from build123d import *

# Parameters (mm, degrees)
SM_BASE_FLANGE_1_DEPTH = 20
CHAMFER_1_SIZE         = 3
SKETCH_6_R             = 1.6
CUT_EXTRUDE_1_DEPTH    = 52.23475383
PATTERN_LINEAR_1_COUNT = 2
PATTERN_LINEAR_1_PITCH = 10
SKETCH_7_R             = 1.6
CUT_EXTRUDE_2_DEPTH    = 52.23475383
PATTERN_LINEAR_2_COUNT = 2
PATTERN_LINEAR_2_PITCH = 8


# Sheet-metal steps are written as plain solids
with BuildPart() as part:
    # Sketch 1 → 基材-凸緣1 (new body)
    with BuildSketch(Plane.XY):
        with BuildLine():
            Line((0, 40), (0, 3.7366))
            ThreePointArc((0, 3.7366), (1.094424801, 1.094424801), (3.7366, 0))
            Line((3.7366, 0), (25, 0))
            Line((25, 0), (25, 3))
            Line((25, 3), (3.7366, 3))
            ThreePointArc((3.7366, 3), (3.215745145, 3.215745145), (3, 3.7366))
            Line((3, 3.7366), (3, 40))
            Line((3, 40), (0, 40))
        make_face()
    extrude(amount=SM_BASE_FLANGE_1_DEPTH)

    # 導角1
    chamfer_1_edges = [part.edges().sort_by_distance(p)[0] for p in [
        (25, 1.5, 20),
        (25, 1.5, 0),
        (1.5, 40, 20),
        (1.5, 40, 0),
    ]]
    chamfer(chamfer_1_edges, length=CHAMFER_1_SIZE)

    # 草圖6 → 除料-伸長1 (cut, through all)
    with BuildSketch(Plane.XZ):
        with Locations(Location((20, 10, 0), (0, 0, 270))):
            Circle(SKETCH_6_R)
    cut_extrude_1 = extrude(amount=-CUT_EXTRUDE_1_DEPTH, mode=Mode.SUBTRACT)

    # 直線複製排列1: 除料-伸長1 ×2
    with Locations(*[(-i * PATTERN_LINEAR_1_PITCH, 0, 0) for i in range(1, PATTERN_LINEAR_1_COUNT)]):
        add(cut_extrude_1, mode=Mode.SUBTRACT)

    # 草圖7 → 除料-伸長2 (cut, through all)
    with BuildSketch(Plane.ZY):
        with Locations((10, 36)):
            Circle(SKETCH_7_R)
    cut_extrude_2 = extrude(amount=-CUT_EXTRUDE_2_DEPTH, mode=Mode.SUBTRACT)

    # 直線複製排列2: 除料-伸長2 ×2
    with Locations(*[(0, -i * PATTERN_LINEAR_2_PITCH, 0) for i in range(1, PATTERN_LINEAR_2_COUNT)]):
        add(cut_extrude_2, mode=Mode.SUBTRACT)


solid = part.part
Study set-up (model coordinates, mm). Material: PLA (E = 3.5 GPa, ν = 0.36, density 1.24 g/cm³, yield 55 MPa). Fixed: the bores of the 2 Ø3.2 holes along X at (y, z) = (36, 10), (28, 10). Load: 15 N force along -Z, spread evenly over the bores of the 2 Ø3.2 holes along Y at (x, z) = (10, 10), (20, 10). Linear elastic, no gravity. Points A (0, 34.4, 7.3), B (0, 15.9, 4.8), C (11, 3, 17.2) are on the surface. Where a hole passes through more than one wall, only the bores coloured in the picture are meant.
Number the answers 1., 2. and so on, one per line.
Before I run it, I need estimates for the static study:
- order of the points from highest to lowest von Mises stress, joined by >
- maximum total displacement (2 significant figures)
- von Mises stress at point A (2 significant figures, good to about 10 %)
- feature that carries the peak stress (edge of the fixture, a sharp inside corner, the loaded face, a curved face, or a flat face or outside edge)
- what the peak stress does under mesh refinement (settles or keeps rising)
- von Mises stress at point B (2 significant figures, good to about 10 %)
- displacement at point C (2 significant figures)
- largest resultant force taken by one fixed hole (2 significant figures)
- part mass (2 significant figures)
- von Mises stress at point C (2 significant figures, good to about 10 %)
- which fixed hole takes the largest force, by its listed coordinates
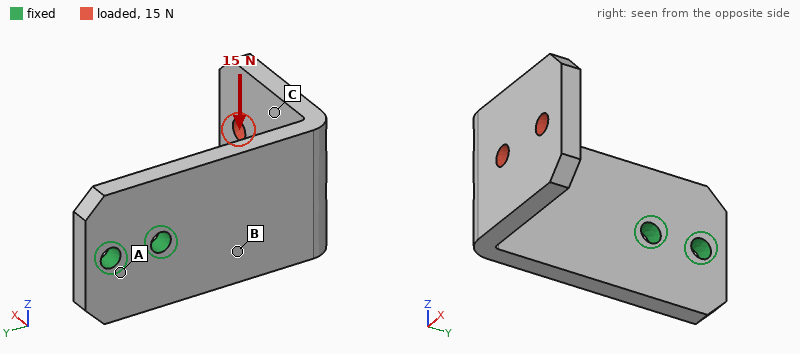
1. B > A > C
2. 0.60 mm
3. 3.1 MPa
4. edge of the fixture
5. keeps rising
6. 5.3 MPa
7. 0.30 mm
8. 47 N
9. 4.4 g
10. 1.2 MPa
11. (28, 10)
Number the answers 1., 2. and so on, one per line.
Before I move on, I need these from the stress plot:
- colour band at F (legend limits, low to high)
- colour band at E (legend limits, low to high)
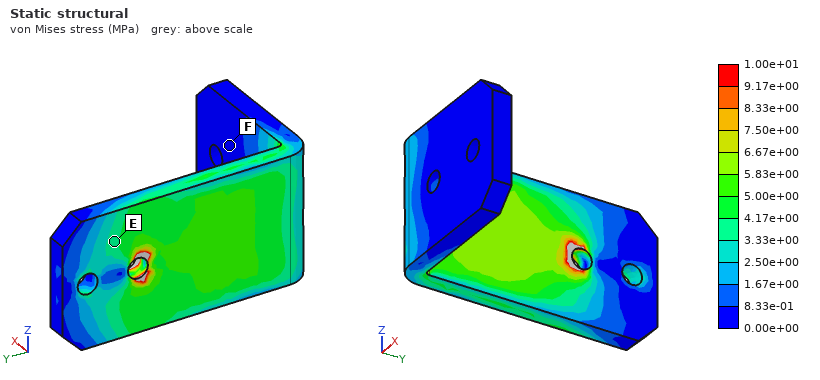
1. 0.00e+00 to 8.33e-01 MPa
2. 3.33e+00 to 4.17e+00 MPa
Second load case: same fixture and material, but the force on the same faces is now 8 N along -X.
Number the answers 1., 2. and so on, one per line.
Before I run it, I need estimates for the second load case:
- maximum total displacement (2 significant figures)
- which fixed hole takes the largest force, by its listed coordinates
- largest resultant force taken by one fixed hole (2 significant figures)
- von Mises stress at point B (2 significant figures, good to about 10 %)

1. 0.53 mm
2. (28, 10)
3. 17 N
4. 3.6 MPa
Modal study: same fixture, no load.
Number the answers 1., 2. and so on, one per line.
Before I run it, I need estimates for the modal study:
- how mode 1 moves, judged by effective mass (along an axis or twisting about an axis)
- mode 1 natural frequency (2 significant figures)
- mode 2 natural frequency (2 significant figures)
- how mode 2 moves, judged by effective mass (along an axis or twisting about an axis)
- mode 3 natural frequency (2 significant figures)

1. along X
2. 460 Hz
3. 760 Hz
4. along Z
5. 1300 Hz
